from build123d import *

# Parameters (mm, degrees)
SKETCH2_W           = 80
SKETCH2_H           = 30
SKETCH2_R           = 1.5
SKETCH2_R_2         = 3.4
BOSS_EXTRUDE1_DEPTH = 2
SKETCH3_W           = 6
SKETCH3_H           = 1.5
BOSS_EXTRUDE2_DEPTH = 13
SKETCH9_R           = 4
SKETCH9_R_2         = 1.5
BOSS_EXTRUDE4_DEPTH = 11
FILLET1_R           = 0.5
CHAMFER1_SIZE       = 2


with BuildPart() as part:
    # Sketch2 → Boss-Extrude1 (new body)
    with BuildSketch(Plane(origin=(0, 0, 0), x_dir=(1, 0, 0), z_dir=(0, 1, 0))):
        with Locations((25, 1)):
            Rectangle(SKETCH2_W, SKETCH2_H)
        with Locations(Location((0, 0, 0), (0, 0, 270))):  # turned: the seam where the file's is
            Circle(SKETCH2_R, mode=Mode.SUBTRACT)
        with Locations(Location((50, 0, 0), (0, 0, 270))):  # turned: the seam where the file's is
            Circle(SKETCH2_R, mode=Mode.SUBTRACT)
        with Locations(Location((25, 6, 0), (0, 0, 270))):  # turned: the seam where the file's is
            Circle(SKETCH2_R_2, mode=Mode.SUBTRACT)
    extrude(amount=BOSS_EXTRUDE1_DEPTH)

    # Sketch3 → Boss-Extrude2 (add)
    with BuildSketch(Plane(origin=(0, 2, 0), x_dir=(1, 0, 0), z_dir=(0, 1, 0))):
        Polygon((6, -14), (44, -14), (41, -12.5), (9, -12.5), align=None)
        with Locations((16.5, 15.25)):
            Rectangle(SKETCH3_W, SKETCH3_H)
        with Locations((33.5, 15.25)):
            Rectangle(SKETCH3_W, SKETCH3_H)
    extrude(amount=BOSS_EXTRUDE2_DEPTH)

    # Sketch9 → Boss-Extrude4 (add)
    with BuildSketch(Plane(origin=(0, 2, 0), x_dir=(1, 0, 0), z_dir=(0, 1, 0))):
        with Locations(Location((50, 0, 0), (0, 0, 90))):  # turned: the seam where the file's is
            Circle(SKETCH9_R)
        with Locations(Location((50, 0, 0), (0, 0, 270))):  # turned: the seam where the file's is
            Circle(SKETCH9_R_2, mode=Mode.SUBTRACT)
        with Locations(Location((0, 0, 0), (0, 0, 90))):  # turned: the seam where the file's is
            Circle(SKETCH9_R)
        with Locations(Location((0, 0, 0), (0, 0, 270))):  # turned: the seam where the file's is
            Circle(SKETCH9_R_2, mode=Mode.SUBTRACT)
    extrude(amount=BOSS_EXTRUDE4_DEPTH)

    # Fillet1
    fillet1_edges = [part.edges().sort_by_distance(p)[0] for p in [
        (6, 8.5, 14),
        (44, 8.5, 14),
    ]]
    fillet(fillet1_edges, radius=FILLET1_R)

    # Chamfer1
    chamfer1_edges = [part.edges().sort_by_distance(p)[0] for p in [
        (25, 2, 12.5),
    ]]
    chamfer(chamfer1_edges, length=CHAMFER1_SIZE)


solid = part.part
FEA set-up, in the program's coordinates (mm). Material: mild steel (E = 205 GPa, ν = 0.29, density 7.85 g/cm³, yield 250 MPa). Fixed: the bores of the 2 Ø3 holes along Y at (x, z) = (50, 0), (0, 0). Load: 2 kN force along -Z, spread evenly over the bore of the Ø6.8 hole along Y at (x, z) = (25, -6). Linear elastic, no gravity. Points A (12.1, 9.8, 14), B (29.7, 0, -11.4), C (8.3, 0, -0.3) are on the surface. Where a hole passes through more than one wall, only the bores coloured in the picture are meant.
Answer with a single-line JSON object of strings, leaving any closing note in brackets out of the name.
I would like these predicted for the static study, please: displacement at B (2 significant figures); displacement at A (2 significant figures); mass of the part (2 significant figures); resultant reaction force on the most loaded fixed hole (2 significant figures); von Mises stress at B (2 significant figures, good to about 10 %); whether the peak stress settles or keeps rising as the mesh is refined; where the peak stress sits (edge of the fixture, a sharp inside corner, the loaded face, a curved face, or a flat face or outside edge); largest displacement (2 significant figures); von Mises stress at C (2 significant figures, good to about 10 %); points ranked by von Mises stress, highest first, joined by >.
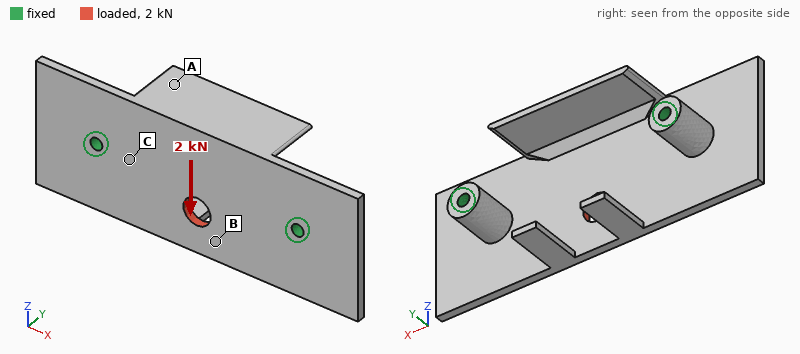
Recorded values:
{"displacement at B": "9.8 µm", "displacement at A": "6.7 µm", "mass of the part": "52 g", "resultant reaction force on the most loaded fixed hole": "1.0 kN", "von Mises stress at B": "55 MPa", "whether the peak stress settles or keeps rising as the mesh is refined": "keeps rising", "where the peak stress sits": "edge of the fixture", "largest displacement": "11 µm", "von Mises stress at C": "37 MPa", "points ranked by von Mises stress, highest first, joined by >": "B > C > A"}
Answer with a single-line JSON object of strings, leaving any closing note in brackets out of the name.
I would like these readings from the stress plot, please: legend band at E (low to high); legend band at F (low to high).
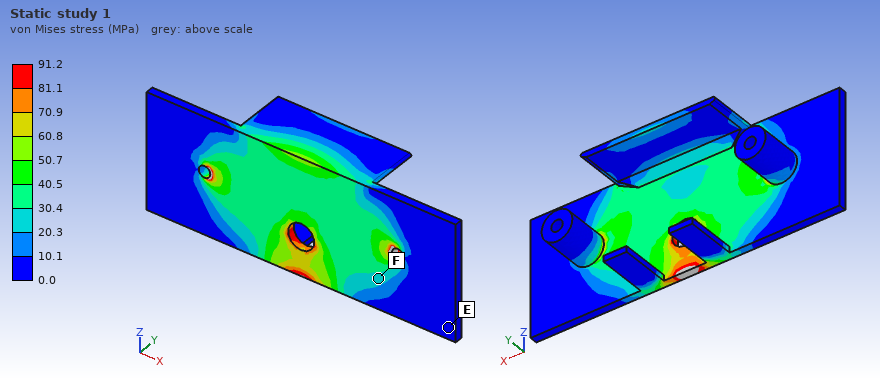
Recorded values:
{"legend band at E": "0.0 to 10.1 MPa", "legend band at F": "20.3 to 30.4 MPa"}
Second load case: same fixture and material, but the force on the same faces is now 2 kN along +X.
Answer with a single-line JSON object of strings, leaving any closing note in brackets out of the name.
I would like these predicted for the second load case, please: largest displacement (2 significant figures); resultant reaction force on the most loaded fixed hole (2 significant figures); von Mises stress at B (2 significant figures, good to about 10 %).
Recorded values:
{"largest displacement": "4.7 µm", "resultant reaction force on the most loaded fixed hole": "1.0 kN", "von Mises stress at B": "23 MPa"}
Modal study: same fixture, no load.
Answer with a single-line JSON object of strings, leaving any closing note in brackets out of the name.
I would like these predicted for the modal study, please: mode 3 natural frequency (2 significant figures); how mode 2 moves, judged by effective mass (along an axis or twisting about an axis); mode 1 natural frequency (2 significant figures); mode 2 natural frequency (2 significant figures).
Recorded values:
{"mode 3 natural frequency": "5400 Hz", "how mode 2 moves, judged by effective mass": "along Y", "mode 1 natural frequency": "3200 Hz", "mode 2 natural frequency": "4000 Hz"}
